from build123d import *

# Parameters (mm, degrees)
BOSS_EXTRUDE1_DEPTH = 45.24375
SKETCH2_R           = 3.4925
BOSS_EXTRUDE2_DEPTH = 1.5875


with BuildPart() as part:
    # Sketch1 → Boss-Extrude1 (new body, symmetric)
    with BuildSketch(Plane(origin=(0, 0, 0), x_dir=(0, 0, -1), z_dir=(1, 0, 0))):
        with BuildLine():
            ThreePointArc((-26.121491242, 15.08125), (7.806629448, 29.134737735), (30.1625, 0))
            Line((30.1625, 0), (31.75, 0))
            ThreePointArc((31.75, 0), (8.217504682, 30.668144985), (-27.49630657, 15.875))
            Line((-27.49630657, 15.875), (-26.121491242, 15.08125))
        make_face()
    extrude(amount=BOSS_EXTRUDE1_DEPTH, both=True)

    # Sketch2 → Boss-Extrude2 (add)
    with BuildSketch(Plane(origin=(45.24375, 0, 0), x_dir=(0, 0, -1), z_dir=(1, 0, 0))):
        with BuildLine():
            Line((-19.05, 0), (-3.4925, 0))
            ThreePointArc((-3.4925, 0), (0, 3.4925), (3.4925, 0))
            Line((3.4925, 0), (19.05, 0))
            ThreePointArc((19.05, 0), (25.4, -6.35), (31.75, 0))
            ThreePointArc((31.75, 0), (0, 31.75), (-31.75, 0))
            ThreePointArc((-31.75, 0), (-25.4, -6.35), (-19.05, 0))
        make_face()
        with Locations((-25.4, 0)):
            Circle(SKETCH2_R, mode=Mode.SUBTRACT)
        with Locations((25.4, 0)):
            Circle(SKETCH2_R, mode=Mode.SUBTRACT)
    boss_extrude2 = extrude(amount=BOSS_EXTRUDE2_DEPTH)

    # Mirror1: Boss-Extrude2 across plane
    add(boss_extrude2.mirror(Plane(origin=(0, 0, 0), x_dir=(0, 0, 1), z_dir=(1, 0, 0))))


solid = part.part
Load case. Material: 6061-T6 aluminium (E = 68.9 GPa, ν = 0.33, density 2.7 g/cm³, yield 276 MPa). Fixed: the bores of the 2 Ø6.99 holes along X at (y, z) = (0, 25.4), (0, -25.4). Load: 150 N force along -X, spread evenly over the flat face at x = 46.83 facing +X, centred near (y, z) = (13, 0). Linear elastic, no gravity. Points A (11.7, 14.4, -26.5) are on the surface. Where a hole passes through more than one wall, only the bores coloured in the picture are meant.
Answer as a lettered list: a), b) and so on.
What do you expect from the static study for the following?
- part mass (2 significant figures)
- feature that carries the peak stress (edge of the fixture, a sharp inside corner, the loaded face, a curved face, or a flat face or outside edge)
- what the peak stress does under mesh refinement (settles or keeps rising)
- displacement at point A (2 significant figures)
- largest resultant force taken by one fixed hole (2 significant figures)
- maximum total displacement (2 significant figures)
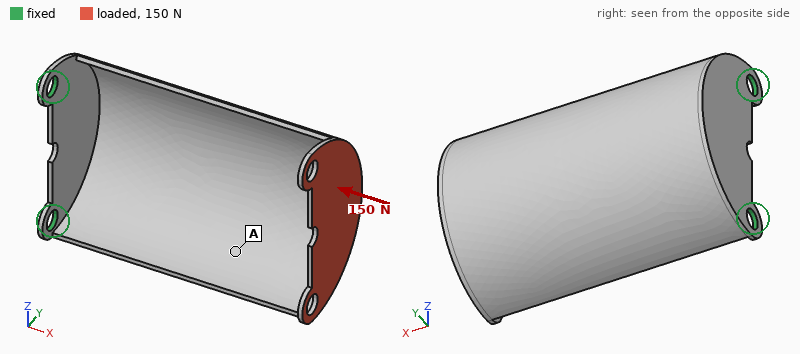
a) 45 g
b) edge of the fixture
c) keeps rising
d) 0.18 mm
e) 76 N
f) 0.50 mm
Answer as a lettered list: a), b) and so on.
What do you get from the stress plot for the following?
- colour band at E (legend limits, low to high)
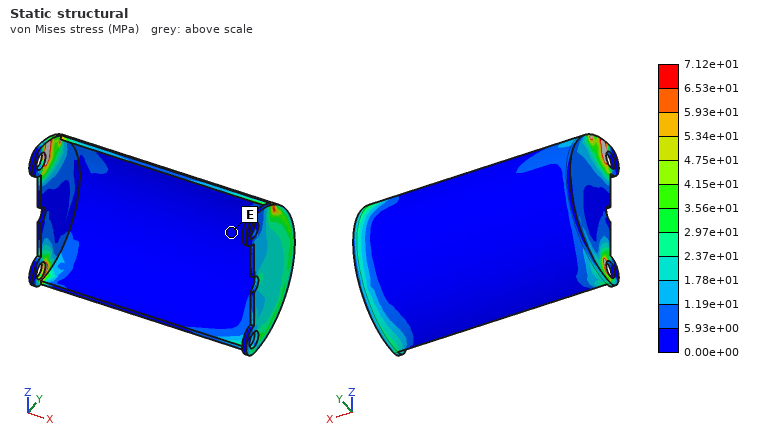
a) 0.00e+00 to 5.93e+00 MPa
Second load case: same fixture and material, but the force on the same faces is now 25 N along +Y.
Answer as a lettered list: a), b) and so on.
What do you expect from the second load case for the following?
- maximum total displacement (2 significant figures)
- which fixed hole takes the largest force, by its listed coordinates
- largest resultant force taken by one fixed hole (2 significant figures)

a) 1.3 mm
b) (0, 25.4)
c) 38 N
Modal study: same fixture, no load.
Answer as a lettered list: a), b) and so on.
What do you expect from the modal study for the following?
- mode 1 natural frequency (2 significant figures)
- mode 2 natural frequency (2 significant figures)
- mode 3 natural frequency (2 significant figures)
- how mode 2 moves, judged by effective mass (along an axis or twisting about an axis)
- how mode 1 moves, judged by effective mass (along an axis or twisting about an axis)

a) 190 Hz
b) 270 Hz
c) 840 Hz
d) along Z
e) along Y
